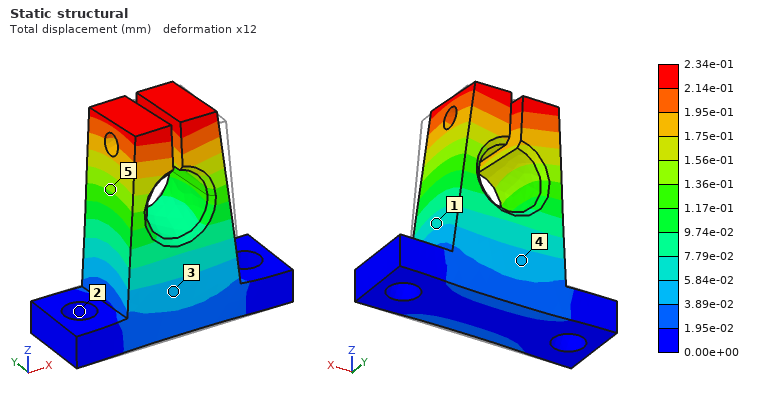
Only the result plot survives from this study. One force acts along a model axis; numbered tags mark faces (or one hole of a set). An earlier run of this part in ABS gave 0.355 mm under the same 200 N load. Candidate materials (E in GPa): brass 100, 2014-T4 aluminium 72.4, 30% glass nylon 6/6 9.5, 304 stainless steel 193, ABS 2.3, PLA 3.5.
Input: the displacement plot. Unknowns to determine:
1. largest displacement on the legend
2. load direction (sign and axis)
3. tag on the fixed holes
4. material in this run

2.34e-01 mm
+Y
2
PLA
